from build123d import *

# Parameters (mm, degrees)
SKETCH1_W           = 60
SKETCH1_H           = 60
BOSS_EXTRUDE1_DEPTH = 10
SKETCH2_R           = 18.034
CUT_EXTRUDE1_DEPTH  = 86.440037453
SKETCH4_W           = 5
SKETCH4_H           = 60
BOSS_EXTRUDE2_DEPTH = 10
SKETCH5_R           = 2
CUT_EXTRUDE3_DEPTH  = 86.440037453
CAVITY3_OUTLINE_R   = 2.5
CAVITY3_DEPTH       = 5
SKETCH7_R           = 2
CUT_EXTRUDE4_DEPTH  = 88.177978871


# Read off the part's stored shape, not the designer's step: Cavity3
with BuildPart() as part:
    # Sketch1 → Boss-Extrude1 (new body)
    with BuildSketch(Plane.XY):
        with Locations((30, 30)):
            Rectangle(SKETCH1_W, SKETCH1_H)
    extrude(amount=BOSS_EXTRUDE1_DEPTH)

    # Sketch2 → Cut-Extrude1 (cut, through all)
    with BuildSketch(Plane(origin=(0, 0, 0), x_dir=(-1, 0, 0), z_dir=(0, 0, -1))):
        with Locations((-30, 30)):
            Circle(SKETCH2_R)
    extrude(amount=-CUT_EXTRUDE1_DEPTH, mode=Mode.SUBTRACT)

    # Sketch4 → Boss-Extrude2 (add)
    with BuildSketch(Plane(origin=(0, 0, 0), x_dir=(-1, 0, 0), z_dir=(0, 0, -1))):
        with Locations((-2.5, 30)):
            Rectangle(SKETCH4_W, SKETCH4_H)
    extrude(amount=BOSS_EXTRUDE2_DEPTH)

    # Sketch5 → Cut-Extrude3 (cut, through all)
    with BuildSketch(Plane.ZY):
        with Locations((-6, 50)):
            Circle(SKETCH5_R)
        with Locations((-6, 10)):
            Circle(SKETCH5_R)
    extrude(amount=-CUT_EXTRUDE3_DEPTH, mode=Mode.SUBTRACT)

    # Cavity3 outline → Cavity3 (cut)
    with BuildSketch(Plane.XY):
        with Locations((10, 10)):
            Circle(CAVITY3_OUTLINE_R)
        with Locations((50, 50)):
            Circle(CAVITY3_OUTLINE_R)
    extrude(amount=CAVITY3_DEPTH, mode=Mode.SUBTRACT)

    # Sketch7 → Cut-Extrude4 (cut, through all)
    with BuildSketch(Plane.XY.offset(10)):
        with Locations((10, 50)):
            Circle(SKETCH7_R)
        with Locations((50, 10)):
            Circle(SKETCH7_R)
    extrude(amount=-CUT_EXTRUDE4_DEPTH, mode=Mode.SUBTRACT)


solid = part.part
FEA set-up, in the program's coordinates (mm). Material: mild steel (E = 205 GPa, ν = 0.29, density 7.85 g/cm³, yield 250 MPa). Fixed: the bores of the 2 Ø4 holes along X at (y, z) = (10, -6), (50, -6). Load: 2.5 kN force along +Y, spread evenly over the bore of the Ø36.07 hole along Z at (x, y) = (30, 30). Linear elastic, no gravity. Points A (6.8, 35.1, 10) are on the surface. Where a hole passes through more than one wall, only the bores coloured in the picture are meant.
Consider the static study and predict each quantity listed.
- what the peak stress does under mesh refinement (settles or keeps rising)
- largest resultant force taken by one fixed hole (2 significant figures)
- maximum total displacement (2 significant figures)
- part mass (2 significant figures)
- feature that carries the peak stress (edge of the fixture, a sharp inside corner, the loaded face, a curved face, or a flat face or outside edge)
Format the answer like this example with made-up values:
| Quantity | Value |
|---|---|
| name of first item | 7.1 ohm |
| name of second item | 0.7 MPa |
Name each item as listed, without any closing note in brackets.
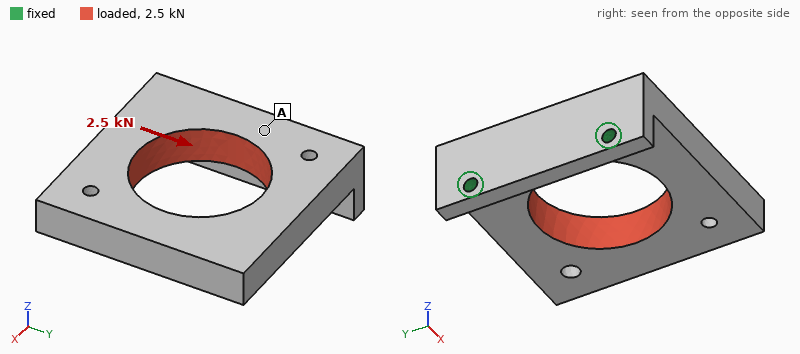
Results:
| Quantity | Value |
|---|---|
| what the peak stress does under mesh refinement | keeps rising |
| largest resultant force taken by one fixed hole | 2.1 kN |
| maximum total displacement | 41 µm |
| part mass | 220 g |
| feature that carries the peak stress | edge of the fixture |
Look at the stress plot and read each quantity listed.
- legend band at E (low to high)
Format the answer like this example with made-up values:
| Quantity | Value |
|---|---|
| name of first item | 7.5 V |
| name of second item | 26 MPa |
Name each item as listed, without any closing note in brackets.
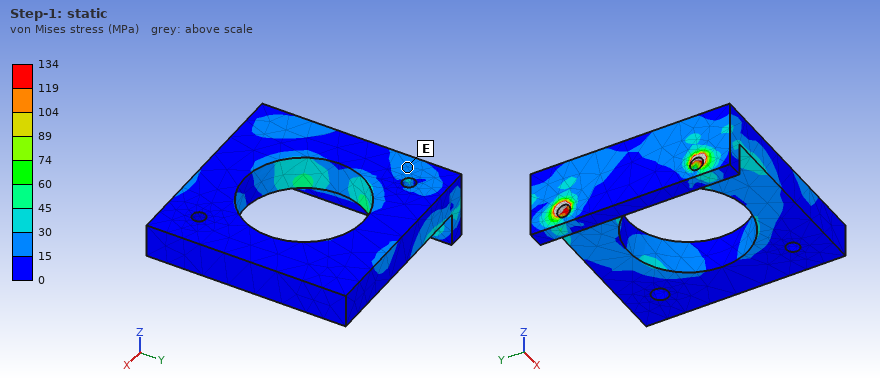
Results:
| Quantity | Value |
|---|---|
| legend band at E | 15 to 30 MPa |
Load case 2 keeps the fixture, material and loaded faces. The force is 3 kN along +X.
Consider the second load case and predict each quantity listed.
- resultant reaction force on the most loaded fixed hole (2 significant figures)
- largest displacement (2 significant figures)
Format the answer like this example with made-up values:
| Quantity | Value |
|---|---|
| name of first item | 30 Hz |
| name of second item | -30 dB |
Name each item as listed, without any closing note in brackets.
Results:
| Quantity | Value |
|---|---|
| resultant reaction force on the most loaded fixed hole | 1.5 kN |
| largest displacement | 0.12 mm |
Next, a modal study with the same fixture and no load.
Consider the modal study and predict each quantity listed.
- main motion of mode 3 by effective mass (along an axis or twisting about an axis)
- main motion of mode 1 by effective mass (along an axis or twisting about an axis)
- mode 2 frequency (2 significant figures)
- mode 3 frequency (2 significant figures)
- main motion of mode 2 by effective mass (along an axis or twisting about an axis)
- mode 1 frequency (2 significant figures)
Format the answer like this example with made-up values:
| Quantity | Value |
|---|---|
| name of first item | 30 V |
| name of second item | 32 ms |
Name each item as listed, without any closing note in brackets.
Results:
| Quantity | Value |
|---|---|
| main motion of mode 3 by effective mass | along Y |
| main motion of mode 1 by effective mass | along Z |
| mode 2 frequency | 2900 Hz |
| mode 3 frequency | 4000 Hz |
| main motion of mode 2 by effective mass | along Y |
| mode 1 frequency | 950 Hz |
